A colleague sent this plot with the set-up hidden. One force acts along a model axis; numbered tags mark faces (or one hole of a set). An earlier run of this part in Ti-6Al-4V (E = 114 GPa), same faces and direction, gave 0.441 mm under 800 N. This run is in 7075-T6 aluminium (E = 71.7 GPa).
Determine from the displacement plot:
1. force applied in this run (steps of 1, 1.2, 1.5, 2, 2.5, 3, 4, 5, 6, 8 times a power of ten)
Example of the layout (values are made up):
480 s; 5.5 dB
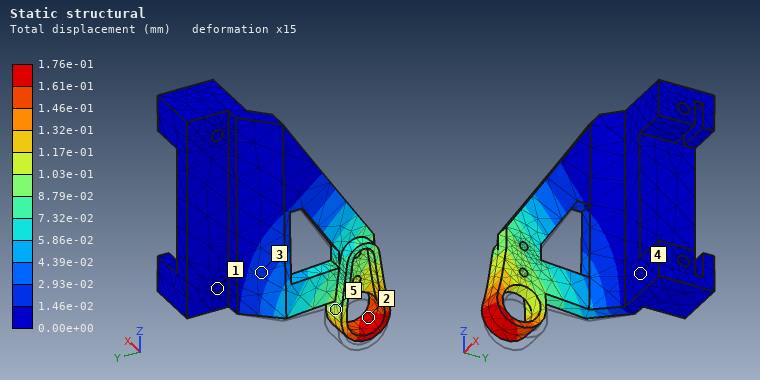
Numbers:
200 N
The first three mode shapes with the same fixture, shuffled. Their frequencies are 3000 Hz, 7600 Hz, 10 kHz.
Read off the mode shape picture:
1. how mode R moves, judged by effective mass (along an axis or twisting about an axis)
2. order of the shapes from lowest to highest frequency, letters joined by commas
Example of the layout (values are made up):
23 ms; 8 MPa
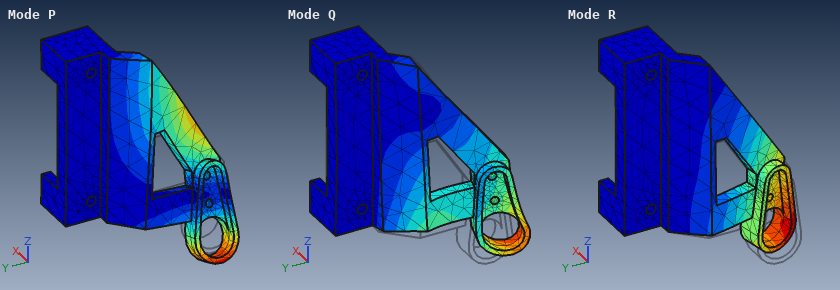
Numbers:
along X; R, P, Q
